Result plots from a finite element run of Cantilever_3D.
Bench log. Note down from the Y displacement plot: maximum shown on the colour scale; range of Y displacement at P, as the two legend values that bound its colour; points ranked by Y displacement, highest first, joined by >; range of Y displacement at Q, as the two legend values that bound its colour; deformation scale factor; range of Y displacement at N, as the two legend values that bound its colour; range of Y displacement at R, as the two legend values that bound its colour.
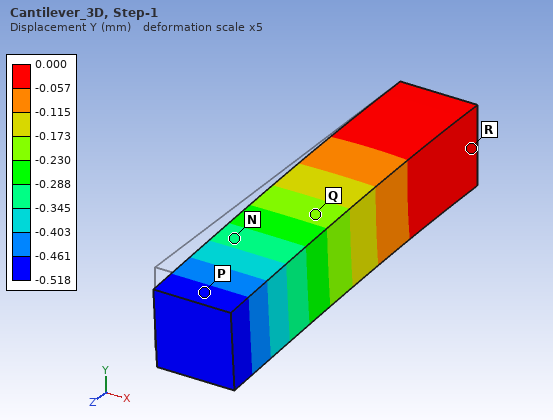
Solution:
0.000 mm
-0.518 to -0.461 mm
R > Q > N > P
-0.230 to -0.173 mm
5
-0.345 to -0.288 mm
-0.057 to 0.000 mm
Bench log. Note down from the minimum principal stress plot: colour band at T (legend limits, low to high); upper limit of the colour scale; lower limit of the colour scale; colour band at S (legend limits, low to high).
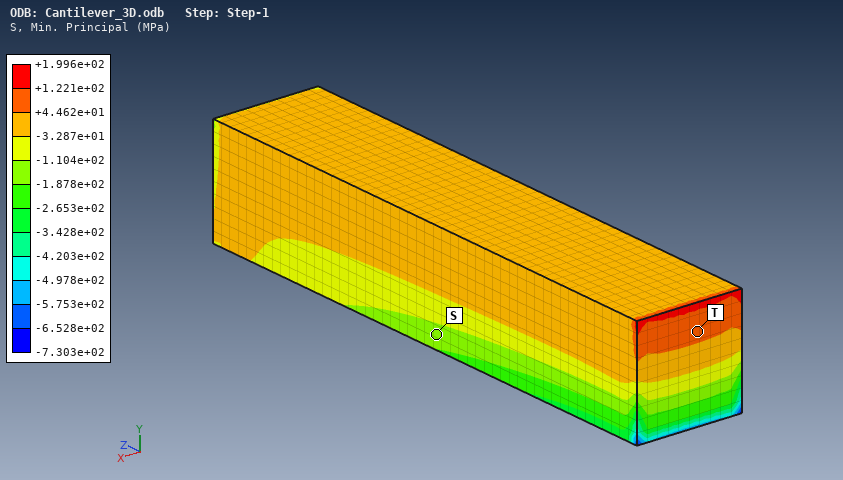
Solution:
+4.462e+01 to +1.221e+02 MPa
+1.996e+02 MPa
-7.303e+02 MPa
-1.878e+02 to -1.104e+02 MPa
